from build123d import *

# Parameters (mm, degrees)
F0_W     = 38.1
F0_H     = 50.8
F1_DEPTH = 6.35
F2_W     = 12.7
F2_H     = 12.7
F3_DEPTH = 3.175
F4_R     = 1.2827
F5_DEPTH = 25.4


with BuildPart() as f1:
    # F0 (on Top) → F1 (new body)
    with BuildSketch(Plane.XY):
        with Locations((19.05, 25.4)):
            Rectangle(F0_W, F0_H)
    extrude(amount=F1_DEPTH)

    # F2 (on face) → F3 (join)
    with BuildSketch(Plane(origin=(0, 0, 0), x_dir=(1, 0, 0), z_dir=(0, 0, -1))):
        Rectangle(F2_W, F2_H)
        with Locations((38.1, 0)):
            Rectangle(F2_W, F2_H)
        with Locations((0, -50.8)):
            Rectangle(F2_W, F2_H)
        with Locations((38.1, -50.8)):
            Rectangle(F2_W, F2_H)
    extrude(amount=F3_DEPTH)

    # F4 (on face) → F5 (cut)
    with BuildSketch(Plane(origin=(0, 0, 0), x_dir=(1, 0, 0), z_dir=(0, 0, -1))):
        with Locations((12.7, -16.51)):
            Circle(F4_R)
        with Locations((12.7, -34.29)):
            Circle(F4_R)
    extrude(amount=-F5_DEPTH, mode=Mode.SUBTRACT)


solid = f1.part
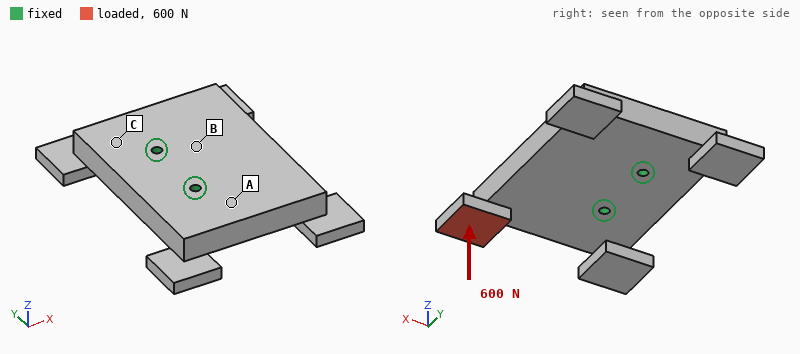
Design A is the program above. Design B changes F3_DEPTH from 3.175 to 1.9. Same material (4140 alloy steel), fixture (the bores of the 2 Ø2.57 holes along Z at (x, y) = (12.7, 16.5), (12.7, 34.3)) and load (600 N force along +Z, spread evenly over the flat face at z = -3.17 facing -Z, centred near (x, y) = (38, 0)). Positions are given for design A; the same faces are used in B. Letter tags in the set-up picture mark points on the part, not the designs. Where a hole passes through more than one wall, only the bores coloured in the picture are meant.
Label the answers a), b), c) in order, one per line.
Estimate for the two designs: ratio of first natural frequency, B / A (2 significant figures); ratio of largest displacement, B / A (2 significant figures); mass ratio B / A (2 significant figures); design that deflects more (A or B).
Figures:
a) 1.1
b) 1.2
c) 0.94
d) B
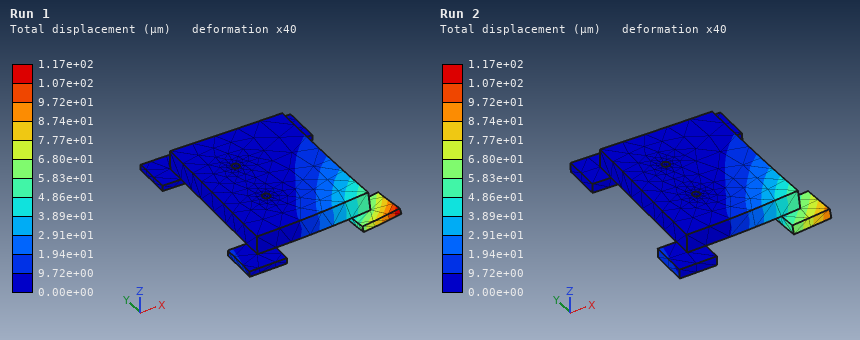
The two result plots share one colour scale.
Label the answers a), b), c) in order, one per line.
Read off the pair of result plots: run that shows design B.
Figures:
a) Run 1
